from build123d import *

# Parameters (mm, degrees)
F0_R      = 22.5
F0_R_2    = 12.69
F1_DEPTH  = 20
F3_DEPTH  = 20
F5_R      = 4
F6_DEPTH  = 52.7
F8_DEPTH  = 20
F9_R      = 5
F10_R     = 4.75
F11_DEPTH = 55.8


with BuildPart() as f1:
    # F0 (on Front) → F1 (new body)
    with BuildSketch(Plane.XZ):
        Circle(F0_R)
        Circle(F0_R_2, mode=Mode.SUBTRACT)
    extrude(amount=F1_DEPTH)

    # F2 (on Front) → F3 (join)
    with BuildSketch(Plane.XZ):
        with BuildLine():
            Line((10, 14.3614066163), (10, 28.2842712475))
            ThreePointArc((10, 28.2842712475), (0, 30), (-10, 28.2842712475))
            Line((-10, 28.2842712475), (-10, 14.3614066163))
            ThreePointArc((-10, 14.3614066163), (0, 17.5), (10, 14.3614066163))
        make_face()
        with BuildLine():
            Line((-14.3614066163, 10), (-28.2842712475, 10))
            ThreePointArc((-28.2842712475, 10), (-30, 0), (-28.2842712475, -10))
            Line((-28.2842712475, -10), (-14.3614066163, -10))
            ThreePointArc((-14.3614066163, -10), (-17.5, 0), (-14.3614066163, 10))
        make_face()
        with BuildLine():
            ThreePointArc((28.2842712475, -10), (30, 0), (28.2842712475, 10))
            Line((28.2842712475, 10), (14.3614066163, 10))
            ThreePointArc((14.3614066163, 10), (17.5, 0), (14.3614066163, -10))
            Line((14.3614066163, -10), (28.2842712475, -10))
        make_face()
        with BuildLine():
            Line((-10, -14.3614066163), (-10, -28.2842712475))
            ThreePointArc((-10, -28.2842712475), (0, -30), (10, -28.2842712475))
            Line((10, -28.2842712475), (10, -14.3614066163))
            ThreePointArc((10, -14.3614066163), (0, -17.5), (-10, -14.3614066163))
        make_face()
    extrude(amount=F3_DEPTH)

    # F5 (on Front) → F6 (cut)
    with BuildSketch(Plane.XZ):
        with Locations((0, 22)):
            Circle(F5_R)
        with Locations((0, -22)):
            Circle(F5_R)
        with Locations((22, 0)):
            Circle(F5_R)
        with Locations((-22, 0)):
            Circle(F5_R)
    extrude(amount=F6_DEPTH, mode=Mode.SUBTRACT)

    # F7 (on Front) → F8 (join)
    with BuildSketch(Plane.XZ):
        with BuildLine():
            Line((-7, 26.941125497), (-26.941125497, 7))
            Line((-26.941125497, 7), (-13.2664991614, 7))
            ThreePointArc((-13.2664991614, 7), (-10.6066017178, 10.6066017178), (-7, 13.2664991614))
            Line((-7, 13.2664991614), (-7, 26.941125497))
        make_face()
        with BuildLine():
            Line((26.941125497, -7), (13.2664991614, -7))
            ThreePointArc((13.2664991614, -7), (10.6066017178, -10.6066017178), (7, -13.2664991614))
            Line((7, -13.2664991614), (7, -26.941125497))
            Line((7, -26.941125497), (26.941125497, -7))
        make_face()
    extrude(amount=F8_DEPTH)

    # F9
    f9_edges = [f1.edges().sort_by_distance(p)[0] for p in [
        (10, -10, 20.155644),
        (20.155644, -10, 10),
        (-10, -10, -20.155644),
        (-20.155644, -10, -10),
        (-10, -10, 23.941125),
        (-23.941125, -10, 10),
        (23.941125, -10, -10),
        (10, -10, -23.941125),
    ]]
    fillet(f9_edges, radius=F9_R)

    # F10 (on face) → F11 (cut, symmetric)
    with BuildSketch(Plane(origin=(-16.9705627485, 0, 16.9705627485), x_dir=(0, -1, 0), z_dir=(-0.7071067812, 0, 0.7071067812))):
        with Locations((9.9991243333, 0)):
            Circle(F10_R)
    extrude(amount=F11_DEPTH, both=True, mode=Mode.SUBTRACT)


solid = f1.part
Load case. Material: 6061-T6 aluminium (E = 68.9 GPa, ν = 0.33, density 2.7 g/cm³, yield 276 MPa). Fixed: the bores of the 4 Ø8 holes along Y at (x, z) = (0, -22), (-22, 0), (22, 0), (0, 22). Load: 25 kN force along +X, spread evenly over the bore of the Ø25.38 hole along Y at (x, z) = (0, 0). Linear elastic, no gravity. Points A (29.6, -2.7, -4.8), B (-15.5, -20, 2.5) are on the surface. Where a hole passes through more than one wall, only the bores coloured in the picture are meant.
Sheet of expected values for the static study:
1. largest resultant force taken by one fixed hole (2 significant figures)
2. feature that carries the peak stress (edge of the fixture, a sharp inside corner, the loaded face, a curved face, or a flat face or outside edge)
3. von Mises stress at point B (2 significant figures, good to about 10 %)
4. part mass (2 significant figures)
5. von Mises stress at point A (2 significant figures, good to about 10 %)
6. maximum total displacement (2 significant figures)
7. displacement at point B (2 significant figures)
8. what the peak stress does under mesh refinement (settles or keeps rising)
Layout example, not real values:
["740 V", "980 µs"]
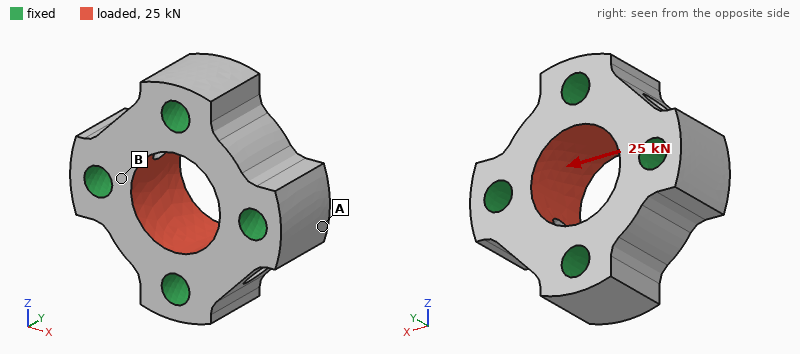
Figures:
["7.2 kN", "edge of the fixture", "28 MPa", "81 g", "7.1 MPa", "6.4 µm", "1.4 µm", "keeps rising"]
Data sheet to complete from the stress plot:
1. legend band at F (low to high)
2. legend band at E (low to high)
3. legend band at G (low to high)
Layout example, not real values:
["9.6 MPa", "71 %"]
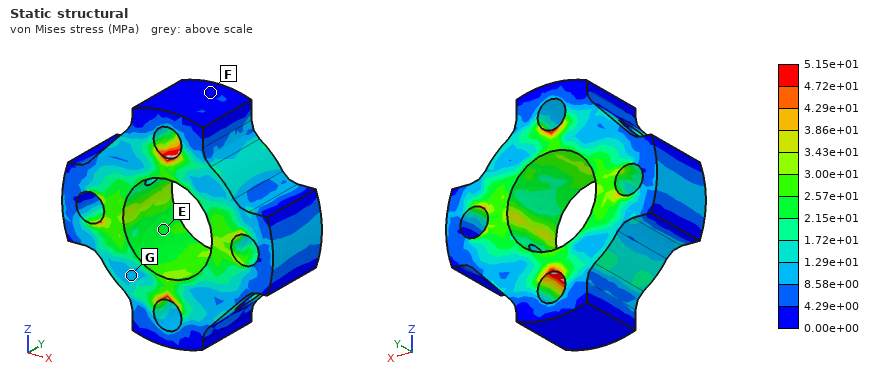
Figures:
["0.00e+00 to 4.29e+00 MPa", "2.15e+01 to 2.57e+01 MPa", "8.58e+00 to 1.29e+01 MPa"]
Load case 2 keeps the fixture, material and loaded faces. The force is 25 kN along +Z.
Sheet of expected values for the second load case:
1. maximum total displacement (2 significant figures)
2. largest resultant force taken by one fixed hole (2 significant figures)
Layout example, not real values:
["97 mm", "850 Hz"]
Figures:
["6.4 µm", "7.1 kN"]
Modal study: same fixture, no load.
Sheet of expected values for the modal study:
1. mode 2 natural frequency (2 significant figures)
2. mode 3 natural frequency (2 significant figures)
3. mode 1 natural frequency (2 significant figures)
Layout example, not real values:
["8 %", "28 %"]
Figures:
["53 kHz", "55 kHz", "47 kHz"]
